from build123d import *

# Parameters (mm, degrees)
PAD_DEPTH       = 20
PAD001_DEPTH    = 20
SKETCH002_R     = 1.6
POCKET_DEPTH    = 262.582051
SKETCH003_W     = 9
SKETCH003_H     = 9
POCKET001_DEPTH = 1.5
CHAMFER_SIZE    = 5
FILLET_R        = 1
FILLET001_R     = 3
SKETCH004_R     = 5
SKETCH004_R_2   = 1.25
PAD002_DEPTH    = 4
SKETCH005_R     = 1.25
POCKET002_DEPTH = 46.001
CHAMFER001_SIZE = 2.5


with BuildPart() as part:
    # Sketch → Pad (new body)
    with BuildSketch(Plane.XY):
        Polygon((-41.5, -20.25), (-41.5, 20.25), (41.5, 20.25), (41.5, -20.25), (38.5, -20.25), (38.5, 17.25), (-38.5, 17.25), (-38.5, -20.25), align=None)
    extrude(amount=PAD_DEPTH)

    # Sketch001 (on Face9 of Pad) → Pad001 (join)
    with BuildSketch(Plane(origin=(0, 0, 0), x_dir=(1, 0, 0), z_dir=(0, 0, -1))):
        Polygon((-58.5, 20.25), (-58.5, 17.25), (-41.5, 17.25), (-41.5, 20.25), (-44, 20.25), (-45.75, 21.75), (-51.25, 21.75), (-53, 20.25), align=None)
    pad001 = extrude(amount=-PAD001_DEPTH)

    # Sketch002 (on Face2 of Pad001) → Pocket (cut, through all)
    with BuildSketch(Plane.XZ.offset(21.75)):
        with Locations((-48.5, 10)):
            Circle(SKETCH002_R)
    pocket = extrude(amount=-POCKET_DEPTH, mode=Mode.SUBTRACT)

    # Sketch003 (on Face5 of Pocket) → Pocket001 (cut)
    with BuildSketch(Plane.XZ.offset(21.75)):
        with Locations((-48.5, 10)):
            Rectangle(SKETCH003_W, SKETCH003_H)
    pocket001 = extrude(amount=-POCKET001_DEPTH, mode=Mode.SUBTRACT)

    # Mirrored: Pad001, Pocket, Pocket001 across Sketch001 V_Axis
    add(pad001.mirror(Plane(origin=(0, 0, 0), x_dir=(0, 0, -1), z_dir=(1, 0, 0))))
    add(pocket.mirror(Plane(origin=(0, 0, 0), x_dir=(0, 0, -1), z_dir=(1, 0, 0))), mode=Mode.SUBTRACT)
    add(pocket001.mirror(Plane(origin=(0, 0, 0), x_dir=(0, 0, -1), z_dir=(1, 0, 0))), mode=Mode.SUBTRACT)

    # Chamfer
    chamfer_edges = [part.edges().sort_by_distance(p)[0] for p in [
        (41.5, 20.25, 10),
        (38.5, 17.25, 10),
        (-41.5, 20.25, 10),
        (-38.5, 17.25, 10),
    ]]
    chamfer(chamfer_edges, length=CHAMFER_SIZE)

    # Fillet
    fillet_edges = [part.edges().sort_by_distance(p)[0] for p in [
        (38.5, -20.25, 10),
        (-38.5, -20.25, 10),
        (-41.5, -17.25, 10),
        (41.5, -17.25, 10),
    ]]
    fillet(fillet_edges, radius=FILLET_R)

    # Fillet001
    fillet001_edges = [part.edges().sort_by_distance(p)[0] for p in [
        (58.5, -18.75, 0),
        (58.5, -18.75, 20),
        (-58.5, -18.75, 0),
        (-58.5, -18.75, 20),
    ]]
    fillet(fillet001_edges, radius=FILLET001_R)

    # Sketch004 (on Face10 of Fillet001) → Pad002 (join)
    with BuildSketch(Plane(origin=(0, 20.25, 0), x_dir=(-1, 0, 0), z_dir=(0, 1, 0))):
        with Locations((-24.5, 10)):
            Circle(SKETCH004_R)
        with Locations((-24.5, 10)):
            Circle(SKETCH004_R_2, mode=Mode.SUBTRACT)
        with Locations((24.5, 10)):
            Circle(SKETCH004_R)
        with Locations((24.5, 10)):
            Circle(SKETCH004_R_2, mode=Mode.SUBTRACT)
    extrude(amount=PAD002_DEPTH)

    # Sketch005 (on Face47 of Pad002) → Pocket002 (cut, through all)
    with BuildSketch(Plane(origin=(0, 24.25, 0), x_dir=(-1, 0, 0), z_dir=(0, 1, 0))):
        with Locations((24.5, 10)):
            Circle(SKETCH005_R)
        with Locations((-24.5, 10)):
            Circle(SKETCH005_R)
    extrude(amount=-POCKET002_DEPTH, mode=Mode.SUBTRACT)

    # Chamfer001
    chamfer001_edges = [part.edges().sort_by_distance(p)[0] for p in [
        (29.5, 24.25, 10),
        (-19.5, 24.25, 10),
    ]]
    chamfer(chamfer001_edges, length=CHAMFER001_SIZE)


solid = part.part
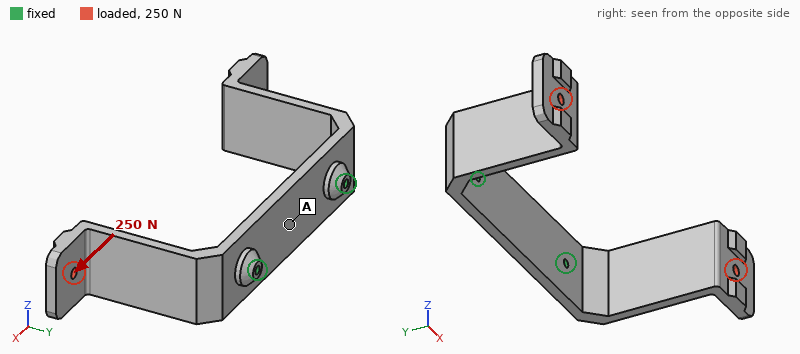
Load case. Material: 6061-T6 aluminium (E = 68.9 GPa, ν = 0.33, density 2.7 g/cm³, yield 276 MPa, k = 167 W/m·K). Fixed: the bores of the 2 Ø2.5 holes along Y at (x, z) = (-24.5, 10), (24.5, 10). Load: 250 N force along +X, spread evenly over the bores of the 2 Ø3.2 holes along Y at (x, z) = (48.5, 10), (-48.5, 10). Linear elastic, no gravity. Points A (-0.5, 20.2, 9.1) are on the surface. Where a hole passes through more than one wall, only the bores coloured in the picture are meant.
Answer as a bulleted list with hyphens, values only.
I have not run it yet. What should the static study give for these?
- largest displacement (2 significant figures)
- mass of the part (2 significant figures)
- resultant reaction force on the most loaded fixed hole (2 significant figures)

- 1.3 mm
- 33 g
- 130 N
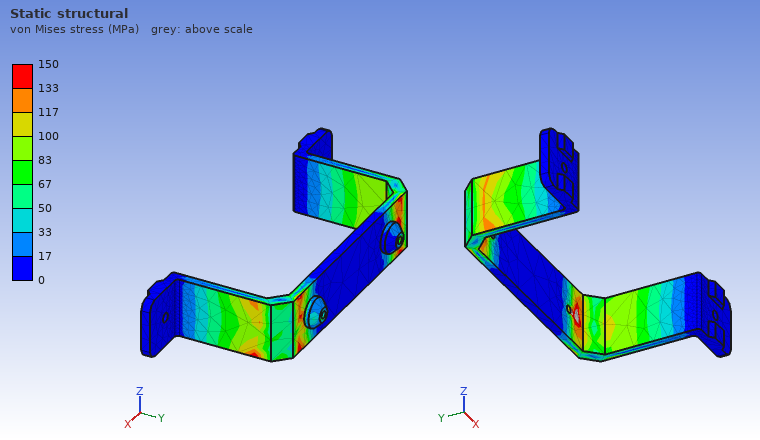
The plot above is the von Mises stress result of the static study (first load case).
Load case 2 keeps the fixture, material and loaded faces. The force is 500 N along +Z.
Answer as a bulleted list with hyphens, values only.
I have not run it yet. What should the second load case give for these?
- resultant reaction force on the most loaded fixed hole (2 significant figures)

- 250 N
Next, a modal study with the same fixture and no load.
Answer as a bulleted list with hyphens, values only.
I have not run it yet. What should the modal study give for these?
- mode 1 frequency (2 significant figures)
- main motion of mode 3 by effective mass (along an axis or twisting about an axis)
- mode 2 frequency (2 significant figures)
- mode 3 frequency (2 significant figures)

- 750 Hz
- along Z
- 750 Hz
- 1400 Hz
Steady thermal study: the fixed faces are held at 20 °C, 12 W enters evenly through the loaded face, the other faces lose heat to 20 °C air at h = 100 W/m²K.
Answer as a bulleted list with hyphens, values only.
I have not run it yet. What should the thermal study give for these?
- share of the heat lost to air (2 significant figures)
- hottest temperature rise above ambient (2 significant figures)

- 55 %
- 21 K
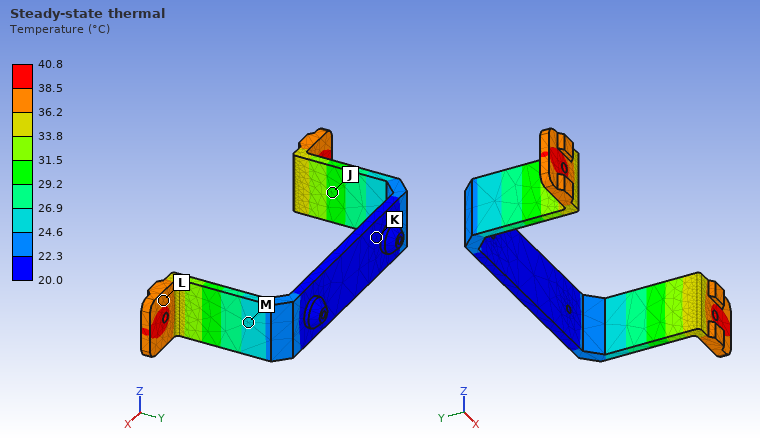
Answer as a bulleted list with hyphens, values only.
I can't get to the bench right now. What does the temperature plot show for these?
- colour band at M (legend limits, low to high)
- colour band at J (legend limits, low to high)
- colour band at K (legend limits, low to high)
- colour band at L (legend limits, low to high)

- 24.6 to 26.9 °C
- 29.2 to 31.5 °C
- 20.0 to 22.3 °C
- 36.2 to 38.5 °C
